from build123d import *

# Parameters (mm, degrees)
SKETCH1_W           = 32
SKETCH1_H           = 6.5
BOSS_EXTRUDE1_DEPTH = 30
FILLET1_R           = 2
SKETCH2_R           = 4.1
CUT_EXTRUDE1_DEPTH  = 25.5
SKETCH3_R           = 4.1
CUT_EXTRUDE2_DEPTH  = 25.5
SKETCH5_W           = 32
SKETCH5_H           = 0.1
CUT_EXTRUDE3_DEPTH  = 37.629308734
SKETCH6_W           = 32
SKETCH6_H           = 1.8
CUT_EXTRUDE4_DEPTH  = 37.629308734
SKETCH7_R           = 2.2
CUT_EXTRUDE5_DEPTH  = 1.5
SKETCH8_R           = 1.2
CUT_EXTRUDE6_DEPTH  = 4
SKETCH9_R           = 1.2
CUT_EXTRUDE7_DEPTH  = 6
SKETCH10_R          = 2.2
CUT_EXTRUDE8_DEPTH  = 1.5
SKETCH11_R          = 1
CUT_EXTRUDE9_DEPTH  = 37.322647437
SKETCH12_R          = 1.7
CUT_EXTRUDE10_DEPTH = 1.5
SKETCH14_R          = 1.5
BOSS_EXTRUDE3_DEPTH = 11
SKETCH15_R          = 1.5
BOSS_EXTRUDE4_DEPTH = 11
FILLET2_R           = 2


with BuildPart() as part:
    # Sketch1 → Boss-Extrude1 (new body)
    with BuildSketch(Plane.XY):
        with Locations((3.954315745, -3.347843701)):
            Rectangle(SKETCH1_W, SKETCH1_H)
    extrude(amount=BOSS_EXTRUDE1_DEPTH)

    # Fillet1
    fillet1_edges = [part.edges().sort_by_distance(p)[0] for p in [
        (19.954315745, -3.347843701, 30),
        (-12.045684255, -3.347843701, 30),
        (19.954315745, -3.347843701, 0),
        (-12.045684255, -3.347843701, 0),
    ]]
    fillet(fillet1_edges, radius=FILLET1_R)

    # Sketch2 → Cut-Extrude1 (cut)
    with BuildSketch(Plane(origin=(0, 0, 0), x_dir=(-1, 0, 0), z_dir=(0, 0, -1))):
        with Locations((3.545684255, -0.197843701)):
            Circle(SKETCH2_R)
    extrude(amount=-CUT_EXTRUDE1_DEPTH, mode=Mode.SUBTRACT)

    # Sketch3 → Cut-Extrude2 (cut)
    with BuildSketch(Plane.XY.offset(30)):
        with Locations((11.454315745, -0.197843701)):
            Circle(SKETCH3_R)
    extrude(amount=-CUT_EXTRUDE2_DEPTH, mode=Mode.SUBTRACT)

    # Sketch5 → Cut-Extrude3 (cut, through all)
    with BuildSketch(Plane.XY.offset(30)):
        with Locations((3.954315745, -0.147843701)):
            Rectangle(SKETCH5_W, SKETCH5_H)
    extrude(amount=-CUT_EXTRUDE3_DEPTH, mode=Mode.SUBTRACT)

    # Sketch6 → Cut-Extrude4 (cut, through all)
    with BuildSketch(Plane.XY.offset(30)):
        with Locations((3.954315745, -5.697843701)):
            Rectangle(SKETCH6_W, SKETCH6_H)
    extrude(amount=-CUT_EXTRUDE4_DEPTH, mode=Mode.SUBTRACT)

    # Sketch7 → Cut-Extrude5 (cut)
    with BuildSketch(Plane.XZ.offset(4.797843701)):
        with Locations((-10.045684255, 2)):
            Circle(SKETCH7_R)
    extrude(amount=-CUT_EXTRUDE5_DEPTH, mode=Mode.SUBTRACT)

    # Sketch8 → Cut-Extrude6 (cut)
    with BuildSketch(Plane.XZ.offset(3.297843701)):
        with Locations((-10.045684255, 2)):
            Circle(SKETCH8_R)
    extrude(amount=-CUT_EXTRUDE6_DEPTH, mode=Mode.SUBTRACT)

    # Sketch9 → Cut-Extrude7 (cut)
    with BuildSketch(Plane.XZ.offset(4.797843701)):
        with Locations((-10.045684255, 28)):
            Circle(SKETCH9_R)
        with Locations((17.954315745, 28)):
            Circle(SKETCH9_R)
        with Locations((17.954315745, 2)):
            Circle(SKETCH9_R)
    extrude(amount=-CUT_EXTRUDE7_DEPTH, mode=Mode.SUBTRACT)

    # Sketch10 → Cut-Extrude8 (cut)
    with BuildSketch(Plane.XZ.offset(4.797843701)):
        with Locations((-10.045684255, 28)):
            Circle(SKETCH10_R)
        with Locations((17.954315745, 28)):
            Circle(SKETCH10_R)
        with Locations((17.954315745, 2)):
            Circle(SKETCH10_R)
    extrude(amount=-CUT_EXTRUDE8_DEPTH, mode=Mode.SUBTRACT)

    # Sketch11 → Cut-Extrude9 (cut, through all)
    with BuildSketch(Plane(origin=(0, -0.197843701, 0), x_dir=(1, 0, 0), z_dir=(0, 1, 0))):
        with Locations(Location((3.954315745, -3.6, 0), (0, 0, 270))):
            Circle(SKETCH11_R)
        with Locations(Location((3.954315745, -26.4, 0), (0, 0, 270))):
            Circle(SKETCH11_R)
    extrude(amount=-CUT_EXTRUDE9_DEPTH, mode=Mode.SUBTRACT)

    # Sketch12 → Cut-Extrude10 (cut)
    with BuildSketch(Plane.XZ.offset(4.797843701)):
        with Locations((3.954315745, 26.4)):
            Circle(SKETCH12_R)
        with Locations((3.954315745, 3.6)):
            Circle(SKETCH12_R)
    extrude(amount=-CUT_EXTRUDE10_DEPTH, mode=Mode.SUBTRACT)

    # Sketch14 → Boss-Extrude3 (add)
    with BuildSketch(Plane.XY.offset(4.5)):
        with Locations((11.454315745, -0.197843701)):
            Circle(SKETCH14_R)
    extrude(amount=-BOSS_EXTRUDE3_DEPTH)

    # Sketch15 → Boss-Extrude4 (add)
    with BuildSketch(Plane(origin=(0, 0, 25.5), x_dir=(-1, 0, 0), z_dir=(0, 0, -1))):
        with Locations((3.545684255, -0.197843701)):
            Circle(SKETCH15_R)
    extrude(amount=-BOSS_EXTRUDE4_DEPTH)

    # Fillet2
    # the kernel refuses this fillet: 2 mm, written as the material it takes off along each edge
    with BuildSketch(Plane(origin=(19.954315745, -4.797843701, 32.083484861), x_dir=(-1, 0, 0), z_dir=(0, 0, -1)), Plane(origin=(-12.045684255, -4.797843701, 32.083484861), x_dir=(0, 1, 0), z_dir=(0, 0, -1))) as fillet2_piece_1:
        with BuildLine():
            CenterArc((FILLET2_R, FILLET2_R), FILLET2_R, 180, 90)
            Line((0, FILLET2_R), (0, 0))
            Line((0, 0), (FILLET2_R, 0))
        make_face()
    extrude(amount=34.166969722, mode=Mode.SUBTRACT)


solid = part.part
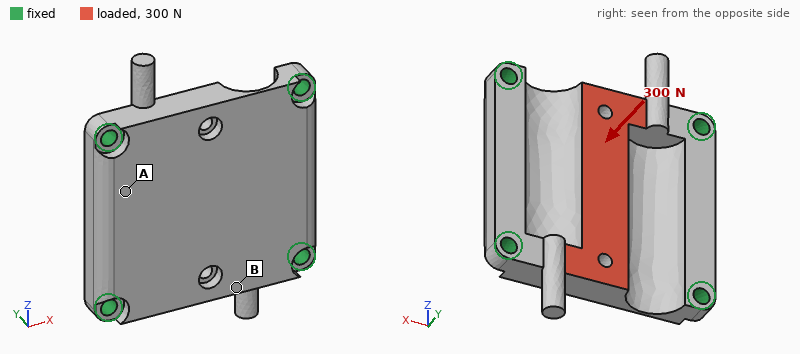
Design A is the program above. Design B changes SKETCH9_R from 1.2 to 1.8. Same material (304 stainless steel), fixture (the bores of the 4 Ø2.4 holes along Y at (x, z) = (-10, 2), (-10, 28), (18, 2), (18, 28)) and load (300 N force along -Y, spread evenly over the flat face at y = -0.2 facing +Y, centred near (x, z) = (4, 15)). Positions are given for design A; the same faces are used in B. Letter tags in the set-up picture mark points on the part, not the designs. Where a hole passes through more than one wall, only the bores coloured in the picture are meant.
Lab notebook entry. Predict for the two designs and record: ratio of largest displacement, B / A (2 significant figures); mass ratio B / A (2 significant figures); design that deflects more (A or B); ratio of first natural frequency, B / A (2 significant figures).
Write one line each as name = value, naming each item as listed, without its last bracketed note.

ratio of largest displacement, B / A = 0.90
mass ratio B / A = 0.98
design that deflects more = A
ratio of first natural frequency, B / A = 1.1
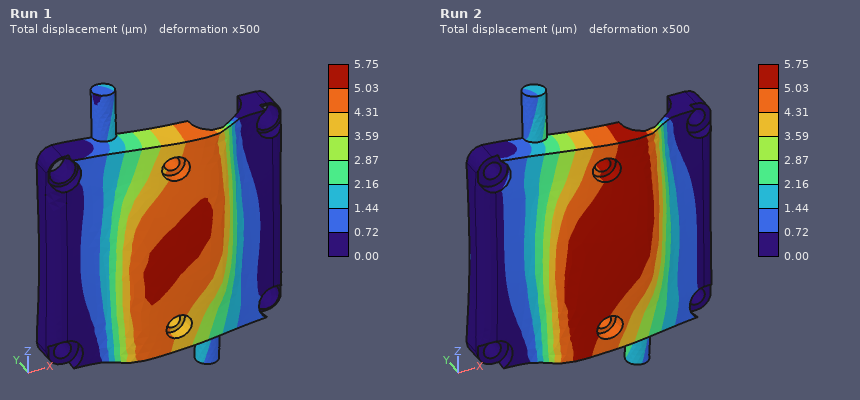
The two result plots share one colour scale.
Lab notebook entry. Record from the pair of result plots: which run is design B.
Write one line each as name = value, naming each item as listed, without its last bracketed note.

which run is design B = Run 1
